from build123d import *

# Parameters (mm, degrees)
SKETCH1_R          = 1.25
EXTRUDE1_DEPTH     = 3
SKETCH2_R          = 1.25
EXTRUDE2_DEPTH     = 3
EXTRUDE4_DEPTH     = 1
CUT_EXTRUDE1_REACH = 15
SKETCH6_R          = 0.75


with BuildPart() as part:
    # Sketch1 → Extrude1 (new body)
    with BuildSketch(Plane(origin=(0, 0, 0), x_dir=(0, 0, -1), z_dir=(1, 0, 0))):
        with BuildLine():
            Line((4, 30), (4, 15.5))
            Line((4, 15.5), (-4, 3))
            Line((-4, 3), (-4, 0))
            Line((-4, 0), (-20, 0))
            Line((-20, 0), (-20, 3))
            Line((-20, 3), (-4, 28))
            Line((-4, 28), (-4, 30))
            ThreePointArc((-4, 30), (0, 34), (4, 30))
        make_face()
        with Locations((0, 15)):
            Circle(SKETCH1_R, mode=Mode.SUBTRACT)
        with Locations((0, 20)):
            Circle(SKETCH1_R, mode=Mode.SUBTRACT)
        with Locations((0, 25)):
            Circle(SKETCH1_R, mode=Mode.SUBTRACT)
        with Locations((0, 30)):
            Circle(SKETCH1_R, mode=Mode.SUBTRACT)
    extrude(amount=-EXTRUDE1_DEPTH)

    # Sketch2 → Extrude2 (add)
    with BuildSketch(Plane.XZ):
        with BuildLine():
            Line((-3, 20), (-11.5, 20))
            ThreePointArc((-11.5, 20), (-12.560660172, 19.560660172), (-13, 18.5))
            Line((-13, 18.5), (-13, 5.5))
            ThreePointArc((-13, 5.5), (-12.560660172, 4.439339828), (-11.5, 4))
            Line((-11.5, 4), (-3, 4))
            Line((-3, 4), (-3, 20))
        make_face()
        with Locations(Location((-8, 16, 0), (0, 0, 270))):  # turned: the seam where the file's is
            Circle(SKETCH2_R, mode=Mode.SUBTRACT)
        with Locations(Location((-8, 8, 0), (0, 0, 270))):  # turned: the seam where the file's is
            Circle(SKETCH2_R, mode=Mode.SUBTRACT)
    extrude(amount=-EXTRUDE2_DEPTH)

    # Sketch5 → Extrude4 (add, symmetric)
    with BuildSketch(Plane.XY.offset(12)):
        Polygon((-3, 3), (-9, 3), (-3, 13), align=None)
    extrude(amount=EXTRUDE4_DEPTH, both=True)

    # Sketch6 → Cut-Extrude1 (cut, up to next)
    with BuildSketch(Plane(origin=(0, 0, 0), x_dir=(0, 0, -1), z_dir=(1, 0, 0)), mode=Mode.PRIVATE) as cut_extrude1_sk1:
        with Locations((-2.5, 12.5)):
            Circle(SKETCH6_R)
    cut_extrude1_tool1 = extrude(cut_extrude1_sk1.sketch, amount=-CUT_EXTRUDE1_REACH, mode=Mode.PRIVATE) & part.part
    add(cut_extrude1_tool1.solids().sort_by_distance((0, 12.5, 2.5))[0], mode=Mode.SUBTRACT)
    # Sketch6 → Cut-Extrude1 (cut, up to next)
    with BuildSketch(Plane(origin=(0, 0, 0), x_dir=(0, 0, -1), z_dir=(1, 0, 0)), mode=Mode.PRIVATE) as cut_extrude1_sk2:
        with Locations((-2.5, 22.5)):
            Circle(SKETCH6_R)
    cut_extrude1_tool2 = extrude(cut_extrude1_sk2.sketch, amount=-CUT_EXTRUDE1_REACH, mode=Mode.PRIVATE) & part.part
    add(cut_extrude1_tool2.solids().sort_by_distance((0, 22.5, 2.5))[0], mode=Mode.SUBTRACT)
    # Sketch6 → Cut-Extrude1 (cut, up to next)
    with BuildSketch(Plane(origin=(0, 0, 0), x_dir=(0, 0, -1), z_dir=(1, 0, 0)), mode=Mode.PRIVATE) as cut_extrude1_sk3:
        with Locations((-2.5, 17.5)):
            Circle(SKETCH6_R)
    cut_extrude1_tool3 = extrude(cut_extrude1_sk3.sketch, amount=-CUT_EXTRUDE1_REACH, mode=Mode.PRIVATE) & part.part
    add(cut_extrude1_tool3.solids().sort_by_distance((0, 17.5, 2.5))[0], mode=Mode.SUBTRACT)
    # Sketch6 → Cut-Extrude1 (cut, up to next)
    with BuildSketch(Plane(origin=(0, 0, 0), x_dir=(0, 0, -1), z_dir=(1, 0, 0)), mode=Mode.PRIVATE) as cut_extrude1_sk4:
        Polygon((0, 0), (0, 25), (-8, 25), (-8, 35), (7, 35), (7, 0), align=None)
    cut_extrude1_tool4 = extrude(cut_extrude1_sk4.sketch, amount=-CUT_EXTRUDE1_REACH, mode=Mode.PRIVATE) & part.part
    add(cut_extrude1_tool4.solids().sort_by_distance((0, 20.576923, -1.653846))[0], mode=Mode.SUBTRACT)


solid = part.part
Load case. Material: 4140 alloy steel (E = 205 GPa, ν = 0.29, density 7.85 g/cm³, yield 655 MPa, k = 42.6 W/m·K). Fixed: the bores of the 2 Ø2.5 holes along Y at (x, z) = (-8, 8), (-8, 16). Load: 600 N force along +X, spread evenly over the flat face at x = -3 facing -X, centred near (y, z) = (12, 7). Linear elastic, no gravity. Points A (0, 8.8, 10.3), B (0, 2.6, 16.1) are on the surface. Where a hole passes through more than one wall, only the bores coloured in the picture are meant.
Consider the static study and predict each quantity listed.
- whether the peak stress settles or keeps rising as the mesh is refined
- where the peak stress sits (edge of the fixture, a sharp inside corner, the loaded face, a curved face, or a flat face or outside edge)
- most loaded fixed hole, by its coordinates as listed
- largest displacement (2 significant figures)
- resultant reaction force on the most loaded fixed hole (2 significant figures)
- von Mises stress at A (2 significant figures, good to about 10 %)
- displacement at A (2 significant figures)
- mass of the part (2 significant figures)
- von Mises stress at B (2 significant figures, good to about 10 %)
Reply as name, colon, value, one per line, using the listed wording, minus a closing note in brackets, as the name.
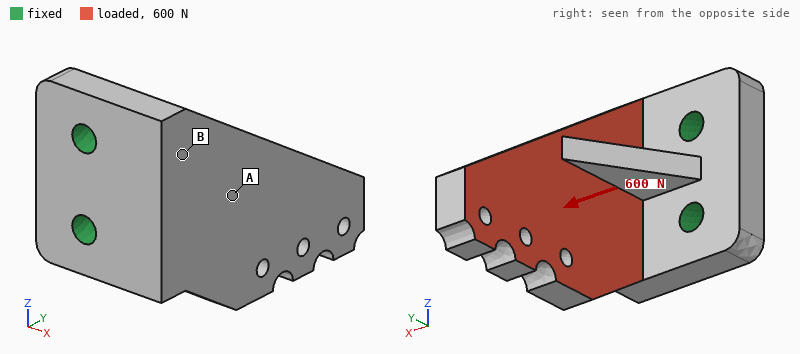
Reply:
whether the peak stress settles or keeps rising as the mesh is refined: keeps rising
where the peak stress sits: edge of the fixture
most loaded fixed hole, by its coordinates as listed: (-8, 8)
largest displacement: 0.15 mm
resultant reaction force on the most loaded fixed hole: 590 N
von Mises stress at A: 130 MPa
displacement at A: 0.030 mm
mass of the part: 11 g
von Mises stress at B: 41 MPa
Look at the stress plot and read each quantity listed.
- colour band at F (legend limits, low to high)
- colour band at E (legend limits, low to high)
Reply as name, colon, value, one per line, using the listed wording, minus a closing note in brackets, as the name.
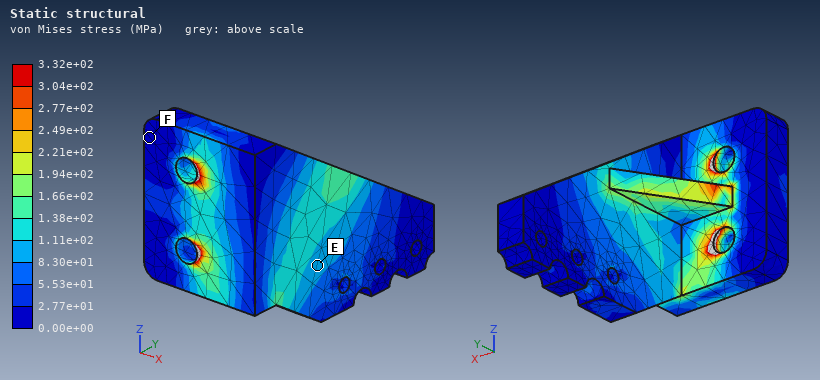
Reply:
colour band at F: 0.00e+00 to 2.77e+01 MPa
colour band at E: 8.30e+01 to 1.11e+02 MPa
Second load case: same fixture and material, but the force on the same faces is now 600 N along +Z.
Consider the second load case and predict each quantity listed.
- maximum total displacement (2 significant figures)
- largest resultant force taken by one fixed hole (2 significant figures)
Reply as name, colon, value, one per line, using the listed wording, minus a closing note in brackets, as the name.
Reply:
maximum total displacement: 47 µm
largest resultant force taken by one fixed hole: 770 N
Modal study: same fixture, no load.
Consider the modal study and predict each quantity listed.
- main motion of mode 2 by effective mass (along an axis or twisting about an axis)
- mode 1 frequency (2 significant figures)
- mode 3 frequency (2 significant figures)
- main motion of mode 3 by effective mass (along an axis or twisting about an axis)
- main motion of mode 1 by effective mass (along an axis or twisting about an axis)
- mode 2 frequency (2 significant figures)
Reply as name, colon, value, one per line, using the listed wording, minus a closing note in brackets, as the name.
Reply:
main motion of mode 2 by effective mass: along Z
mode 1 frequency: 5600 Hz
mode 3 frequency: 18 kHz
main motion of mode 3 by effective mass: along Y
main motion of mode 1 by effective mass: along X
mode 2 frequency: 9600 Hz
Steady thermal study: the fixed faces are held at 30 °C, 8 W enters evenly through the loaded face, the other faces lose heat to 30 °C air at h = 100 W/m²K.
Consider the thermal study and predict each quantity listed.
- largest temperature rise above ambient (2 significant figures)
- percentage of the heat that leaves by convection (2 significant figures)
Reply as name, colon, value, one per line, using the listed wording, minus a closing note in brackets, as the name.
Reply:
largest temperature rise above ambient: 50 K
percentage of the heat that leaves by convection: 27 %
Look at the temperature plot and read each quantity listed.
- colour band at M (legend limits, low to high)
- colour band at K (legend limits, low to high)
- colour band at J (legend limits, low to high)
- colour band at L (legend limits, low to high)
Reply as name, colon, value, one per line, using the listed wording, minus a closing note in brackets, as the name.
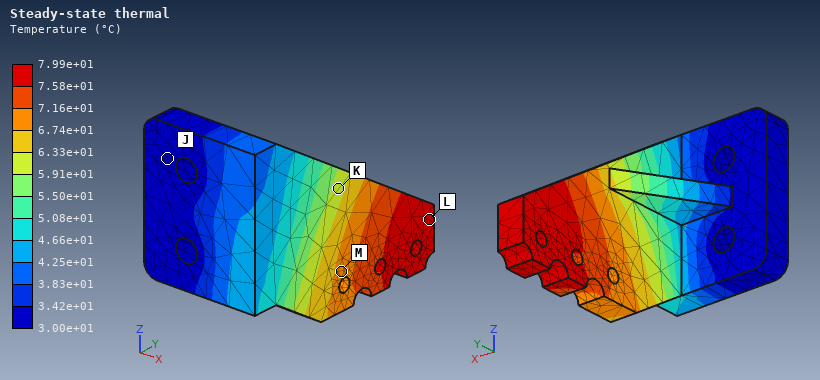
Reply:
colour band at M: 6.74e+01 to 7.16e+01 °C
colour band at K: 5.91e+01 to 6.33e+01 °C
colour band at J: 3.00e+01 to 3.42e+01 °C
colour band at L: 7.58e+01 to 7.99e+01 °C
